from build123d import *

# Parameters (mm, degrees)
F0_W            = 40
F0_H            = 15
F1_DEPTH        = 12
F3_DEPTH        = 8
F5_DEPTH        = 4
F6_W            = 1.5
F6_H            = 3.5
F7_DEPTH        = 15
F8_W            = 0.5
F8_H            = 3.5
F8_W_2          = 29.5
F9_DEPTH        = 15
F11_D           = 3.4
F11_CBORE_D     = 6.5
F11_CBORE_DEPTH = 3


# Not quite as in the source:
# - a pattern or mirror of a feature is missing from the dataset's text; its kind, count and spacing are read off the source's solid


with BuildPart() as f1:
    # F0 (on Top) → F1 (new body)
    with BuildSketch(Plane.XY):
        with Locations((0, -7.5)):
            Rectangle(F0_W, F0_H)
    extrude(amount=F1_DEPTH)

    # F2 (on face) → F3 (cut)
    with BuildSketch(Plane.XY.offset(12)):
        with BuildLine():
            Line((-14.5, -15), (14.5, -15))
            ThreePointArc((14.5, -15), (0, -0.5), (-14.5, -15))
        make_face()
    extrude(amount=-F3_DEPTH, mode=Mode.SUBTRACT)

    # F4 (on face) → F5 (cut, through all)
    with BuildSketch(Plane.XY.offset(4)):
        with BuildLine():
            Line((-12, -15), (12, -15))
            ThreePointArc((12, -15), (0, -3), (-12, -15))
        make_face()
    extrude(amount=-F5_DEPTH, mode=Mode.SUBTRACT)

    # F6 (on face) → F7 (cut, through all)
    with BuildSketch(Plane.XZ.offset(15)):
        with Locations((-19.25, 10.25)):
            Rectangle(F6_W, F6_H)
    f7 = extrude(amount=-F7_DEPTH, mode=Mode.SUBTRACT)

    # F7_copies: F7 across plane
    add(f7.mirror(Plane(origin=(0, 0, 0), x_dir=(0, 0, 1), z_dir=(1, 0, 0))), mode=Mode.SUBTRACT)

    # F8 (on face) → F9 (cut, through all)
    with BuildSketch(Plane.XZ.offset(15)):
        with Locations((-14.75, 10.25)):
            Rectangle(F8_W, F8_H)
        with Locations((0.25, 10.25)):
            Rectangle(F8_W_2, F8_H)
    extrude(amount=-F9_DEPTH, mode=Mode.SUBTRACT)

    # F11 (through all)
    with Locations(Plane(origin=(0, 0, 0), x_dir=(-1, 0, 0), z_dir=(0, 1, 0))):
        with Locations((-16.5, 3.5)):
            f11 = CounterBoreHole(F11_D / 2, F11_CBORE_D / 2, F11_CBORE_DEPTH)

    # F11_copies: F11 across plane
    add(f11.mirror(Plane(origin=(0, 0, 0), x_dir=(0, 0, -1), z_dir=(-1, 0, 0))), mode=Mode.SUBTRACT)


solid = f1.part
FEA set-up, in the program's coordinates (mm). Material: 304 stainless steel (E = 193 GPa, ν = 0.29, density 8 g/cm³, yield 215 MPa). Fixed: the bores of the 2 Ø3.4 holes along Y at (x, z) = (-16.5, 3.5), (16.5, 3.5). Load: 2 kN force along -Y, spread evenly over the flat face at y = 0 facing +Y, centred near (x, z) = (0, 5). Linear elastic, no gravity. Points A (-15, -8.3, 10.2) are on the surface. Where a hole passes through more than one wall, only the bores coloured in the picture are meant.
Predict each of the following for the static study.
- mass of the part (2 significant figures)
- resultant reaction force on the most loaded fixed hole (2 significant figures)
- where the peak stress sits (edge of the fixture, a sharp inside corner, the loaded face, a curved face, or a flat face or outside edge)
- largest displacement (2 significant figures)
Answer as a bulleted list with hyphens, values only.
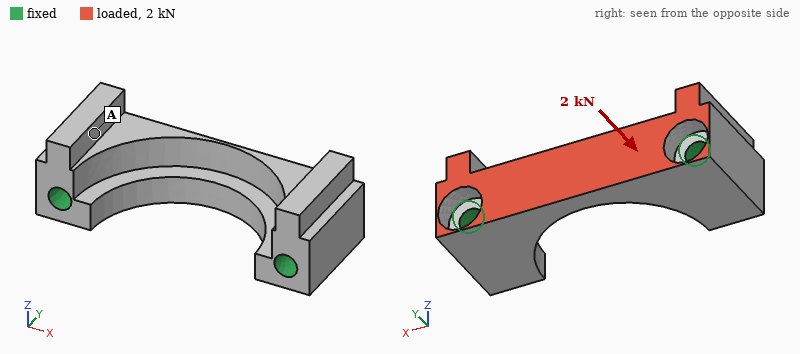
- 21 g
- 1.2 kN
- the loaded face
- 24 µm
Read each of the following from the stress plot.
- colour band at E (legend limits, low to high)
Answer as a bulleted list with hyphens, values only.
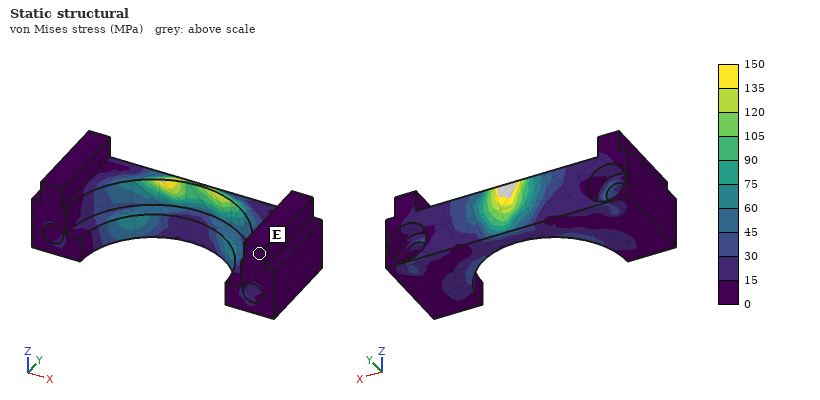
- 0 to 15 MPa
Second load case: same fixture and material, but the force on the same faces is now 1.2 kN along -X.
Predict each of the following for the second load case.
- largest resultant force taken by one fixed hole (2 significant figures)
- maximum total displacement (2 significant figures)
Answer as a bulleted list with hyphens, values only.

- 610 N
- 3.2 µm
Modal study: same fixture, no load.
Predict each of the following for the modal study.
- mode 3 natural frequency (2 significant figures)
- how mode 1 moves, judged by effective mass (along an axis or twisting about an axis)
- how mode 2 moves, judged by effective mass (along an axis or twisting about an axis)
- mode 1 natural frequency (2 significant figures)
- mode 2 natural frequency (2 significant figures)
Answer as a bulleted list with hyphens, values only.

- 46 kHz
- along Z
- along Y
- 30 kHz
- 41 kHz
